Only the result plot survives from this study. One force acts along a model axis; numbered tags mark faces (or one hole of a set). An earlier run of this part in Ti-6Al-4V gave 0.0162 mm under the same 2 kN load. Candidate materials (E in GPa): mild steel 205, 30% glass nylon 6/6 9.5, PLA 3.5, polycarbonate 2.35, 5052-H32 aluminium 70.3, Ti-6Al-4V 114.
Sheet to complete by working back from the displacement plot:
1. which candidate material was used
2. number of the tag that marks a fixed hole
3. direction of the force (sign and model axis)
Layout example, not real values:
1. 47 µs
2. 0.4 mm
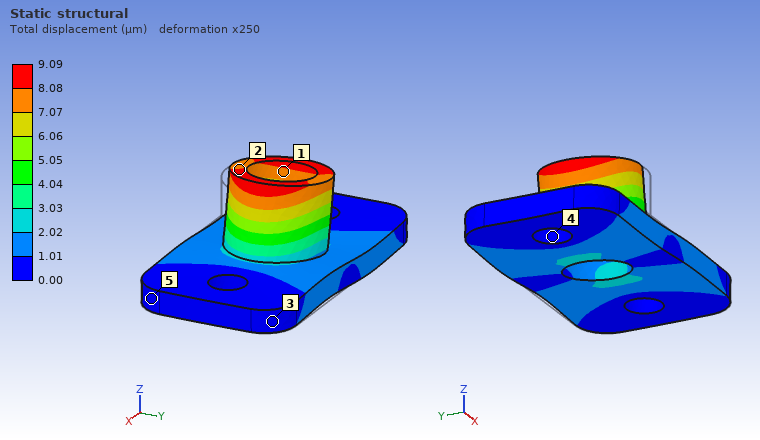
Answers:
1. mild steel
2. 4
3. -X
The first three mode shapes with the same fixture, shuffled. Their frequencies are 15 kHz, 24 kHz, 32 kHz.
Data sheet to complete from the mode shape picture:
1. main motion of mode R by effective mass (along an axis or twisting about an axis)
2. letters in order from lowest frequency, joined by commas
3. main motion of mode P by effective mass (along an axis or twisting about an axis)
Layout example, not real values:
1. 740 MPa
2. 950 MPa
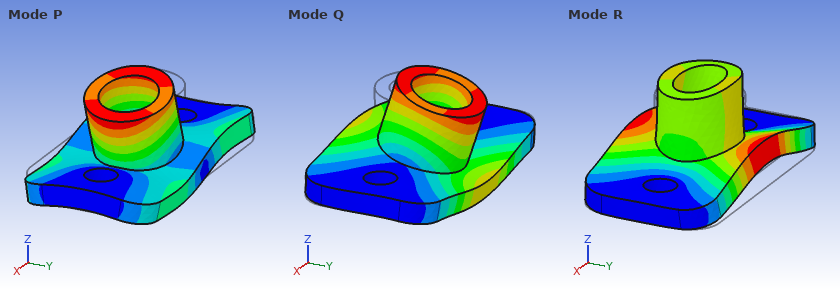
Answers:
1. along Z
2. Q, R, P
3. along X
